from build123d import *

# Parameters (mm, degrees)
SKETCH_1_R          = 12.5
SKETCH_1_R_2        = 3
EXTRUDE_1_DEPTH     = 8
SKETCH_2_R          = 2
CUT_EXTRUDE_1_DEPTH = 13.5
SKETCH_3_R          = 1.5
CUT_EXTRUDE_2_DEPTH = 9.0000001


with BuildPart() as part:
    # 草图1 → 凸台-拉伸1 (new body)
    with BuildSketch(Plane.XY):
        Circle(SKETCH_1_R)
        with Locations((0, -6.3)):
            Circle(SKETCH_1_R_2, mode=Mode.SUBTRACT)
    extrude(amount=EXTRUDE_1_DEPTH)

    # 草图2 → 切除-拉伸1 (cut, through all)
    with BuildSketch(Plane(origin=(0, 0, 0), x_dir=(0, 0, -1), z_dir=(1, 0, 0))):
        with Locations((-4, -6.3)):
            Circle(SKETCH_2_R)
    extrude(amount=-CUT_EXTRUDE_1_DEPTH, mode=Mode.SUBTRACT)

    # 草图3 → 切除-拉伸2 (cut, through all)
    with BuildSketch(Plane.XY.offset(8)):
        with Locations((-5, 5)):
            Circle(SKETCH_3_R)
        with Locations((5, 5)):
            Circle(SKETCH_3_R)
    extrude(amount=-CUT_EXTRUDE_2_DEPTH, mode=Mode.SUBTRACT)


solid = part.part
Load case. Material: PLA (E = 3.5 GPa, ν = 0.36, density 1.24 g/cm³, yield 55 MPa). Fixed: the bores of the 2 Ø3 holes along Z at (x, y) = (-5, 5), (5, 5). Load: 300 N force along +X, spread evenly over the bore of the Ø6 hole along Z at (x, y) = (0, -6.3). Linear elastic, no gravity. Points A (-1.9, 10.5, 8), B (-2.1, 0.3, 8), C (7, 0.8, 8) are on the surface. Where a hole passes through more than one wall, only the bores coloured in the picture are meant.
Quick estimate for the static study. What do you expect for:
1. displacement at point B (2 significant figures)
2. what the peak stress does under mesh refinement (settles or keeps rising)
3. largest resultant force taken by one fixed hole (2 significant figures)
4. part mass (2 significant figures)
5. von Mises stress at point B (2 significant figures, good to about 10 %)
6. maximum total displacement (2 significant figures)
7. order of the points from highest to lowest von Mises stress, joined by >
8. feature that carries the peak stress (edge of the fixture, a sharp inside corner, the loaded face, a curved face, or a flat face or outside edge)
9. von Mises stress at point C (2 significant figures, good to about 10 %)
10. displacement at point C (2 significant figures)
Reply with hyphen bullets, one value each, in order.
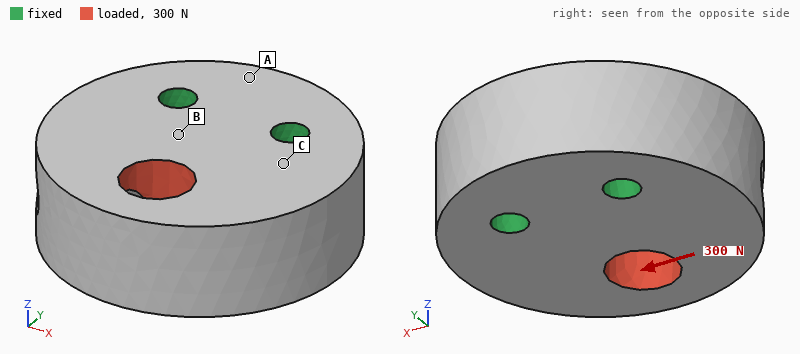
- 10 µm
- keeps rising
- 300 N
- 4.3 g
- 6.0 MPa
- 47 µm
- B > C > A
- edge of the fixture
- 2.7 MPa
- 12 µm
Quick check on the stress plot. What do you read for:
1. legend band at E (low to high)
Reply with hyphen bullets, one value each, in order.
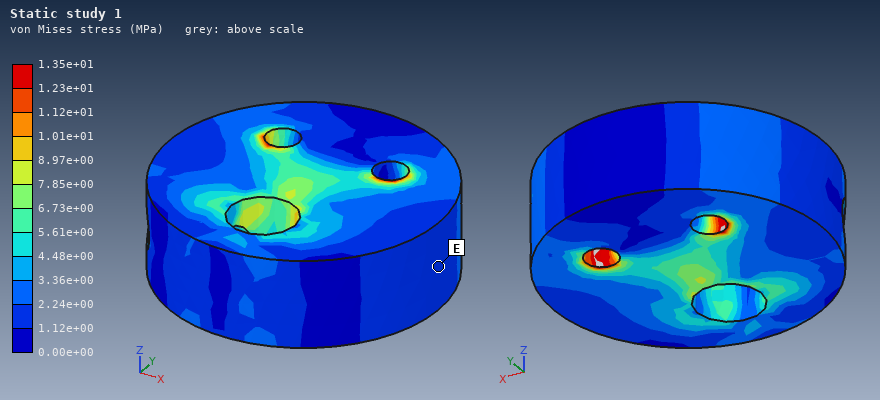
- 1.12e+00 to 2.24e+00 MPa
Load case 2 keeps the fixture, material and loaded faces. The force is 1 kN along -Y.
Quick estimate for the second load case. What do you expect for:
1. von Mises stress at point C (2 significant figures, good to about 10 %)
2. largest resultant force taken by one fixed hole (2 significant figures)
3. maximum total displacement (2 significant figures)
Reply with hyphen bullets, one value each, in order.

- 6.3 MPa
- 540 N
- 61 µm
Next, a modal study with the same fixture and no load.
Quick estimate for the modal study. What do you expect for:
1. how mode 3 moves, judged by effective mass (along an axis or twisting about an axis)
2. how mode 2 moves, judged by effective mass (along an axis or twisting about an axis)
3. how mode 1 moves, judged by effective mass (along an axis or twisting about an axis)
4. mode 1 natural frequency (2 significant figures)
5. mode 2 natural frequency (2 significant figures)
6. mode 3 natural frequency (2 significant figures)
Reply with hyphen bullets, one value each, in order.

- twisting about Y
- along X
- along Z
- 7400 Hz
- 10 kHz
- 12 kHz
